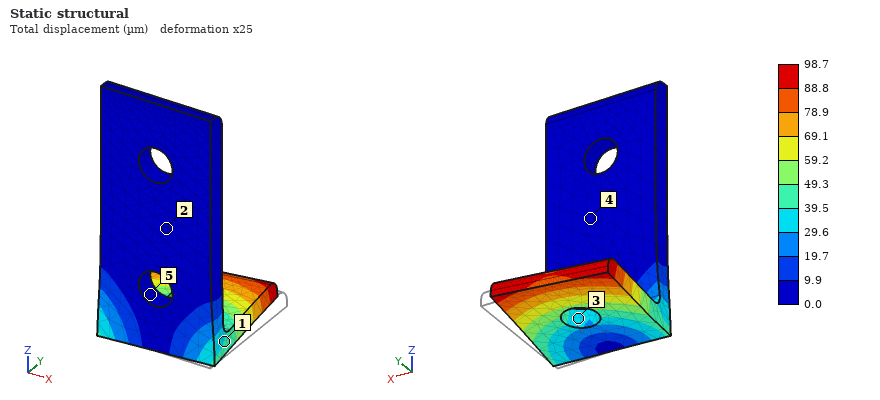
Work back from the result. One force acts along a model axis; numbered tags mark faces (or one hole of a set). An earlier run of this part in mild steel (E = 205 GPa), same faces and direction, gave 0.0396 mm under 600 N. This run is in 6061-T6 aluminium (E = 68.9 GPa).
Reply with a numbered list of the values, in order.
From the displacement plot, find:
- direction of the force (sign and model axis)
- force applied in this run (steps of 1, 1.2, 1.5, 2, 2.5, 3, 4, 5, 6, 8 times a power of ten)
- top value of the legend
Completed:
1. -X
2. 500 N
3. 98.7 µm
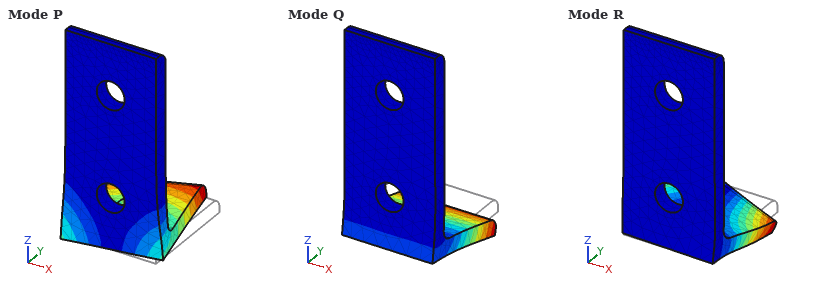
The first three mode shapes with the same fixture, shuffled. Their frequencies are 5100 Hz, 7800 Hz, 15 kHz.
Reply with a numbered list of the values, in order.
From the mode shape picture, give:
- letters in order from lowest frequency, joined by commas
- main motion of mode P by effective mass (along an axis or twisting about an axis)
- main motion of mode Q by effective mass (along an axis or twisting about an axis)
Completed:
1. Q, P, R
2. along X
3. along Z
